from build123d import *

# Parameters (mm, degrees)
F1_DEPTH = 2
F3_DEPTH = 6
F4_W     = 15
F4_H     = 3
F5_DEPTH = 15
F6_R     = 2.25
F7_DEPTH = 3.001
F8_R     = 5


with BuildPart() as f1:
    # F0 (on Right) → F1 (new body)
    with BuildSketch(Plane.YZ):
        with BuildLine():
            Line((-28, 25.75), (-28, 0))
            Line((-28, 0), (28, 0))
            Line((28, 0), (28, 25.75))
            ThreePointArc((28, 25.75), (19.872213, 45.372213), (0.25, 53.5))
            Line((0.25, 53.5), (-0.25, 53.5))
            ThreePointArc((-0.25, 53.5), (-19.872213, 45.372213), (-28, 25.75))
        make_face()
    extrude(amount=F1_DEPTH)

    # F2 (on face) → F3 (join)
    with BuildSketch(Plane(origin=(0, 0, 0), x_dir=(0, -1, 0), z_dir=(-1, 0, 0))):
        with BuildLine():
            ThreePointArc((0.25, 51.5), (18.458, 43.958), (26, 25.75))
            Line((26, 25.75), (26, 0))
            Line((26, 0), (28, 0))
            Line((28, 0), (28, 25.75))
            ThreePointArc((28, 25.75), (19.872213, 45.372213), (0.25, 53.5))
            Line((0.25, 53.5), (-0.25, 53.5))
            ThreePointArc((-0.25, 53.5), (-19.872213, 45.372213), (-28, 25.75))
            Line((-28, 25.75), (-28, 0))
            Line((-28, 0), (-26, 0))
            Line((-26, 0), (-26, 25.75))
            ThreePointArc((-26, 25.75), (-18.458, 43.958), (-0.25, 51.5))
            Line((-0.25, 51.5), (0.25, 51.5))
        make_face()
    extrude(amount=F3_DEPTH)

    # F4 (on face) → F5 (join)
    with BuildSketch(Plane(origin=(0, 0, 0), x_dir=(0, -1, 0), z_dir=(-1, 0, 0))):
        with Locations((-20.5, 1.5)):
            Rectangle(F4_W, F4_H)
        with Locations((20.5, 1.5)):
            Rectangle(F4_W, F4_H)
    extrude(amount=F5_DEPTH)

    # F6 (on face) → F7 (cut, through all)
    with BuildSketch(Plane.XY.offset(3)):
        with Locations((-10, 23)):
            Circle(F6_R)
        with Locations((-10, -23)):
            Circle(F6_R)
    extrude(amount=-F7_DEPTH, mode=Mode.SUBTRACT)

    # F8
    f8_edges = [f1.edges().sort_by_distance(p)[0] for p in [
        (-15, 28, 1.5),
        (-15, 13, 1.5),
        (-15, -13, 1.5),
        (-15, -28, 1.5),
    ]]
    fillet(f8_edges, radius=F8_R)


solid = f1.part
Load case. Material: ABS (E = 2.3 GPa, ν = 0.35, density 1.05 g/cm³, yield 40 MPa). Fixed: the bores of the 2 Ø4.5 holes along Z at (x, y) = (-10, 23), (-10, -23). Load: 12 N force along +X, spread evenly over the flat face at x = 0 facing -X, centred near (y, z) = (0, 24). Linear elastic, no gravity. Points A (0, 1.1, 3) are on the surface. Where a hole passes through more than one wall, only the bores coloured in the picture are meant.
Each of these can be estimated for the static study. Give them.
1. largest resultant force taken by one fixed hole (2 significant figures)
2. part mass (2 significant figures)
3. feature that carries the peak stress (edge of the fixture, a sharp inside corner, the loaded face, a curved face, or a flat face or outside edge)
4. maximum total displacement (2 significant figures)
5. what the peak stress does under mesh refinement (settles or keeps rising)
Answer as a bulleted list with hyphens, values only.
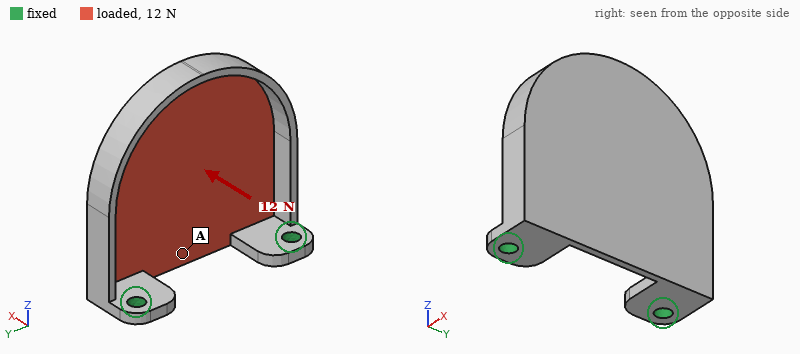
- 6.1 N
- 8.5 g
- edge of the fixture
- 0.89 mm
- keeps rising
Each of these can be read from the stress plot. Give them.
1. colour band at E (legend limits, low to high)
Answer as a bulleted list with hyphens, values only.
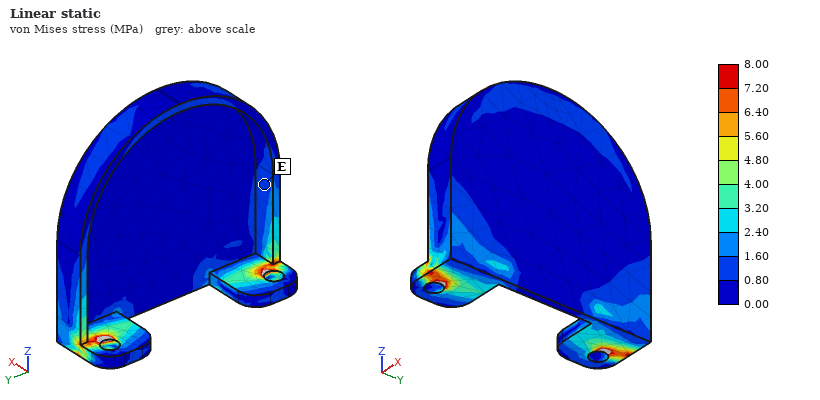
- 0.80 to 1.60 MPa
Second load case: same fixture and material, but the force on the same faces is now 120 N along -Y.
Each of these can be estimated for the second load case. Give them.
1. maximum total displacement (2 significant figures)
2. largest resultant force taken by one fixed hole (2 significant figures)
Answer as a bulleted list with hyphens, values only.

- 0.86 mm
- 81 N
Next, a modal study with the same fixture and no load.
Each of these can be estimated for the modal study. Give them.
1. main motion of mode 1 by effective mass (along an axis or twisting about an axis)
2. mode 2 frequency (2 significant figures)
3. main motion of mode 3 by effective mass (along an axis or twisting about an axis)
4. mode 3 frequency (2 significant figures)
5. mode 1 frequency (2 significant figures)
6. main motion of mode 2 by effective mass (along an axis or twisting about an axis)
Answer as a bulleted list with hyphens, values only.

- along X
- 620 Hz
- along Z
- 1500 Hz
- 260 Hz
- along Y
